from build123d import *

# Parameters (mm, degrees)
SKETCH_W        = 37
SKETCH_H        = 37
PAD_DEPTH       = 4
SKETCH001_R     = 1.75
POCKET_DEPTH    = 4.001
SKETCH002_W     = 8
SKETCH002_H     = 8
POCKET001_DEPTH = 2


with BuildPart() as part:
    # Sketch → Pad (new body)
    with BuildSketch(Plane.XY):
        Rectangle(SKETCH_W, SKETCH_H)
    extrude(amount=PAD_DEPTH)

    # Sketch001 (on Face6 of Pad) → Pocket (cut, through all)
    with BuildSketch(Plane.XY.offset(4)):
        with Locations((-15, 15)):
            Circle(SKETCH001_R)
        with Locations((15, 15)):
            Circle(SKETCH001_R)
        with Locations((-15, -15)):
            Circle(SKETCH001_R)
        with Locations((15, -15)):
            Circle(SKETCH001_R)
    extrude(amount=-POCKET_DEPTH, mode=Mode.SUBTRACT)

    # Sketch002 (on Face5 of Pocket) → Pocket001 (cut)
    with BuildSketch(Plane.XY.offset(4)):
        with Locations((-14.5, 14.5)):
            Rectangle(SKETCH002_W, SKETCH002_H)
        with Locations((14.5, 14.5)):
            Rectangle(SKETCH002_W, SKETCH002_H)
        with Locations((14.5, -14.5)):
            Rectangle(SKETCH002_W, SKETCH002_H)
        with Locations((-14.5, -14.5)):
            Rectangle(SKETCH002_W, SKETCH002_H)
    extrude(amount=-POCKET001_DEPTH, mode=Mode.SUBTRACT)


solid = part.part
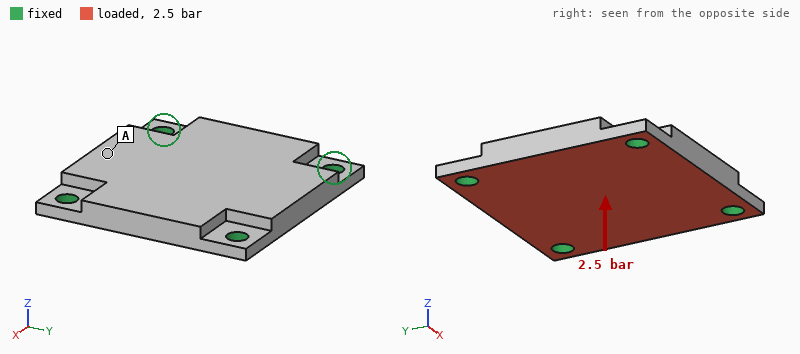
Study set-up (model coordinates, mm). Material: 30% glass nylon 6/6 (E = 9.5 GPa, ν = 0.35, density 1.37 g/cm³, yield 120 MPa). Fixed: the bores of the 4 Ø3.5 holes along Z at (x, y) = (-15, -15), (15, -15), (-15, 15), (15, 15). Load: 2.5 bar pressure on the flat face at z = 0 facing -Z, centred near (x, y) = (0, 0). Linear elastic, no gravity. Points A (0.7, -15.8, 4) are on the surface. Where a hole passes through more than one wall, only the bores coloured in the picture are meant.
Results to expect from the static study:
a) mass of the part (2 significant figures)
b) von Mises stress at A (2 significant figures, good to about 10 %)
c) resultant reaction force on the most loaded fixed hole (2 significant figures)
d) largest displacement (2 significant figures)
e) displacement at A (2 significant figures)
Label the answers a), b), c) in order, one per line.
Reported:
a) 6.7 g
b) 6.6 MPa
c) 110 N
d) 41 µm
e) 25 µm
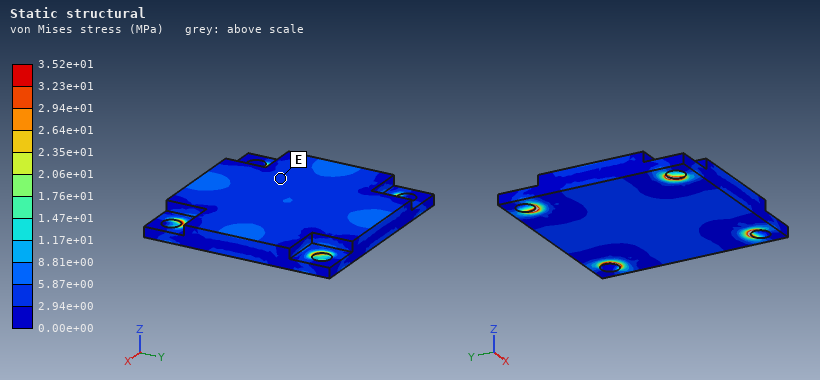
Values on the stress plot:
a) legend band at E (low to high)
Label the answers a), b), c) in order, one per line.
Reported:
a) 2.94e+00 to 5.87e+00 MPa
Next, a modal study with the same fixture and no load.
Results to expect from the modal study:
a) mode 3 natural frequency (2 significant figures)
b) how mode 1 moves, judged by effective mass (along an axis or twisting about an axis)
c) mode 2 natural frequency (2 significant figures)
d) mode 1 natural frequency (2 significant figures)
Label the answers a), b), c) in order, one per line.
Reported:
a) 9900 Hz
b) along Z
c) 9900 Hz
d) 6300 Hz
